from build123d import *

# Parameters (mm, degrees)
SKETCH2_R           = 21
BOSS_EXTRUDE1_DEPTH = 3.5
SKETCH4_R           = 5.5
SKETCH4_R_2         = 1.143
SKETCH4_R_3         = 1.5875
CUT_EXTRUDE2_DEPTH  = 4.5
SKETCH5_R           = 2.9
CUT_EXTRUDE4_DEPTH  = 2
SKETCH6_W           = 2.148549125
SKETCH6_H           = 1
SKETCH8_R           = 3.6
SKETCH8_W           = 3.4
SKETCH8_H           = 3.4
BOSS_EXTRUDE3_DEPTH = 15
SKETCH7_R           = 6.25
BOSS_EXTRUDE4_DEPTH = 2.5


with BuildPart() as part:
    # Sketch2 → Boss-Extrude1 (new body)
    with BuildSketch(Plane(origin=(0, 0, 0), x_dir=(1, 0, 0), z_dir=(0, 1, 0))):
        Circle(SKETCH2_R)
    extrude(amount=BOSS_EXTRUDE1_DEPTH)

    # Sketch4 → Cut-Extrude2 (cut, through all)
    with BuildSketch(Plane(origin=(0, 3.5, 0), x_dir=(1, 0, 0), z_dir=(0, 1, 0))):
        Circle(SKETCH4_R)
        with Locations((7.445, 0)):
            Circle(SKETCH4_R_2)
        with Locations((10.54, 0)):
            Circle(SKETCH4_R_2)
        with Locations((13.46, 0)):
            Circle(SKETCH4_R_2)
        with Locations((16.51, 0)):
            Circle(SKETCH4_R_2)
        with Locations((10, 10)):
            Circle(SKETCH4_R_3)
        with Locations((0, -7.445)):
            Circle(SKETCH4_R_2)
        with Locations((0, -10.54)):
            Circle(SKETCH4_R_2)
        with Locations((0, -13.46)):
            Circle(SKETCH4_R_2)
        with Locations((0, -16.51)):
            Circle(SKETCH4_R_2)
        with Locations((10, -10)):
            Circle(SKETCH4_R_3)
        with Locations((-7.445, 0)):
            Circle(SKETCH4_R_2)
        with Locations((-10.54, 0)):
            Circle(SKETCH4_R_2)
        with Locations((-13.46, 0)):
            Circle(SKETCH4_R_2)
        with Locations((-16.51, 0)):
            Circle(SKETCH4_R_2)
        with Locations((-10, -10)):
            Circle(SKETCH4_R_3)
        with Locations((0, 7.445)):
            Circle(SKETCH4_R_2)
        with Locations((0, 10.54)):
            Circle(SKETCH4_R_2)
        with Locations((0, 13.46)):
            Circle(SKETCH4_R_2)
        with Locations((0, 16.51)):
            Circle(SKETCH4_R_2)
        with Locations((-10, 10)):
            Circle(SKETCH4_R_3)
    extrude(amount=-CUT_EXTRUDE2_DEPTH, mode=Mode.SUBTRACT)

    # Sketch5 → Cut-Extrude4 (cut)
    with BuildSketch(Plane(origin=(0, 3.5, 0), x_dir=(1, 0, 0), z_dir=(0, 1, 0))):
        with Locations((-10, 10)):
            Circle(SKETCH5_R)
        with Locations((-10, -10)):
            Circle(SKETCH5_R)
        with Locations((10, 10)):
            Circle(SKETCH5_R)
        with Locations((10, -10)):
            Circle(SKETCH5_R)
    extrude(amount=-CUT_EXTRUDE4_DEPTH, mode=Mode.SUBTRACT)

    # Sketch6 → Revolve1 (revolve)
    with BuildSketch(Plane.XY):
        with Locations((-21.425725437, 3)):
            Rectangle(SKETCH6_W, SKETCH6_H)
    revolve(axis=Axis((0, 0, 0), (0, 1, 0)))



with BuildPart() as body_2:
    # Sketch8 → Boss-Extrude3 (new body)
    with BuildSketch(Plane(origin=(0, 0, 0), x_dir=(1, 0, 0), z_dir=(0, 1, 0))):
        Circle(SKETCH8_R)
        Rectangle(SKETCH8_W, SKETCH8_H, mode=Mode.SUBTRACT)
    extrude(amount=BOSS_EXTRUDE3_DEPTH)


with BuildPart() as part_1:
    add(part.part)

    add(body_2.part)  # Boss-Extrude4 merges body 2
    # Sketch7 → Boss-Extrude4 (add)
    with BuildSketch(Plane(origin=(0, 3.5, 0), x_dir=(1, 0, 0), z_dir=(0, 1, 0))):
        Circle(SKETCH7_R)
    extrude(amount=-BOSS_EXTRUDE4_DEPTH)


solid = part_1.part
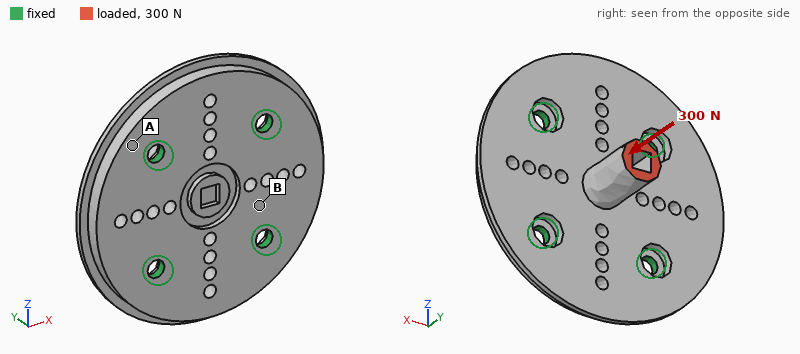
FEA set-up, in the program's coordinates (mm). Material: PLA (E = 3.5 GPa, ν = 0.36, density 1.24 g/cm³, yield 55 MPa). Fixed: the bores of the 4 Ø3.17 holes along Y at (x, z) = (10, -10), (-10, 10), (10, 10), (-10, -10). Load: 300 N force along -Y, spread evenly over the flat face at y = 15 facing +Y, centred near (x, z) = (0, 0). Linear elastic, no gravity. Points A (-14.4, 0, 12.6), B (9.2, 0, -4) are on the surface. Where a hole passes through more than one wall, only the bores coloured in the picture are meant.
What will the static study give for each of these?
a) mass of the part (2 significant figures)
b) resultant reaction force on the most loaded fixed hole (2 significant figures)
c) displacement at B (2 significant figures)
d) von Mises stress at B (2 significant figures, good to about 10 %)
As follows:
6.0 g
150 N
0.053 mm
7.9 MPa
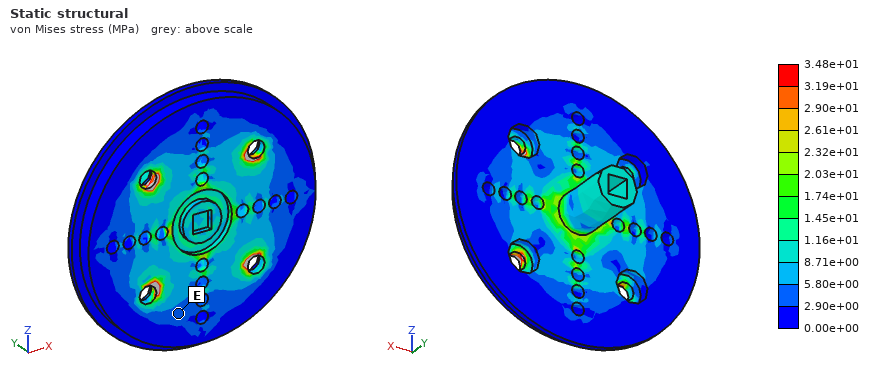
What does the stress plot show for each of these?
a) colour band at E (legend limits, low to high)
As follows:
2.90e+00 to 5.80e+00 MPa
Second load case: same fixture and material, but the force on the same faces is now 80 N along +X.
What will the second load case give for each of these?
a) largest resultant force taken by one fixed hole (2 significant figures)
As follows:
49 N
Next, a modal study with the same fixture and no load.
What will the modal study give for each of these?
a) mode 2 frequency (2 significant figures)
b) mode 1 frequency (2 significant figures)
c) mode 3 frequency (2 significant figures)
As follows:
5400 Hz
4700 Hz
5400 Hz
